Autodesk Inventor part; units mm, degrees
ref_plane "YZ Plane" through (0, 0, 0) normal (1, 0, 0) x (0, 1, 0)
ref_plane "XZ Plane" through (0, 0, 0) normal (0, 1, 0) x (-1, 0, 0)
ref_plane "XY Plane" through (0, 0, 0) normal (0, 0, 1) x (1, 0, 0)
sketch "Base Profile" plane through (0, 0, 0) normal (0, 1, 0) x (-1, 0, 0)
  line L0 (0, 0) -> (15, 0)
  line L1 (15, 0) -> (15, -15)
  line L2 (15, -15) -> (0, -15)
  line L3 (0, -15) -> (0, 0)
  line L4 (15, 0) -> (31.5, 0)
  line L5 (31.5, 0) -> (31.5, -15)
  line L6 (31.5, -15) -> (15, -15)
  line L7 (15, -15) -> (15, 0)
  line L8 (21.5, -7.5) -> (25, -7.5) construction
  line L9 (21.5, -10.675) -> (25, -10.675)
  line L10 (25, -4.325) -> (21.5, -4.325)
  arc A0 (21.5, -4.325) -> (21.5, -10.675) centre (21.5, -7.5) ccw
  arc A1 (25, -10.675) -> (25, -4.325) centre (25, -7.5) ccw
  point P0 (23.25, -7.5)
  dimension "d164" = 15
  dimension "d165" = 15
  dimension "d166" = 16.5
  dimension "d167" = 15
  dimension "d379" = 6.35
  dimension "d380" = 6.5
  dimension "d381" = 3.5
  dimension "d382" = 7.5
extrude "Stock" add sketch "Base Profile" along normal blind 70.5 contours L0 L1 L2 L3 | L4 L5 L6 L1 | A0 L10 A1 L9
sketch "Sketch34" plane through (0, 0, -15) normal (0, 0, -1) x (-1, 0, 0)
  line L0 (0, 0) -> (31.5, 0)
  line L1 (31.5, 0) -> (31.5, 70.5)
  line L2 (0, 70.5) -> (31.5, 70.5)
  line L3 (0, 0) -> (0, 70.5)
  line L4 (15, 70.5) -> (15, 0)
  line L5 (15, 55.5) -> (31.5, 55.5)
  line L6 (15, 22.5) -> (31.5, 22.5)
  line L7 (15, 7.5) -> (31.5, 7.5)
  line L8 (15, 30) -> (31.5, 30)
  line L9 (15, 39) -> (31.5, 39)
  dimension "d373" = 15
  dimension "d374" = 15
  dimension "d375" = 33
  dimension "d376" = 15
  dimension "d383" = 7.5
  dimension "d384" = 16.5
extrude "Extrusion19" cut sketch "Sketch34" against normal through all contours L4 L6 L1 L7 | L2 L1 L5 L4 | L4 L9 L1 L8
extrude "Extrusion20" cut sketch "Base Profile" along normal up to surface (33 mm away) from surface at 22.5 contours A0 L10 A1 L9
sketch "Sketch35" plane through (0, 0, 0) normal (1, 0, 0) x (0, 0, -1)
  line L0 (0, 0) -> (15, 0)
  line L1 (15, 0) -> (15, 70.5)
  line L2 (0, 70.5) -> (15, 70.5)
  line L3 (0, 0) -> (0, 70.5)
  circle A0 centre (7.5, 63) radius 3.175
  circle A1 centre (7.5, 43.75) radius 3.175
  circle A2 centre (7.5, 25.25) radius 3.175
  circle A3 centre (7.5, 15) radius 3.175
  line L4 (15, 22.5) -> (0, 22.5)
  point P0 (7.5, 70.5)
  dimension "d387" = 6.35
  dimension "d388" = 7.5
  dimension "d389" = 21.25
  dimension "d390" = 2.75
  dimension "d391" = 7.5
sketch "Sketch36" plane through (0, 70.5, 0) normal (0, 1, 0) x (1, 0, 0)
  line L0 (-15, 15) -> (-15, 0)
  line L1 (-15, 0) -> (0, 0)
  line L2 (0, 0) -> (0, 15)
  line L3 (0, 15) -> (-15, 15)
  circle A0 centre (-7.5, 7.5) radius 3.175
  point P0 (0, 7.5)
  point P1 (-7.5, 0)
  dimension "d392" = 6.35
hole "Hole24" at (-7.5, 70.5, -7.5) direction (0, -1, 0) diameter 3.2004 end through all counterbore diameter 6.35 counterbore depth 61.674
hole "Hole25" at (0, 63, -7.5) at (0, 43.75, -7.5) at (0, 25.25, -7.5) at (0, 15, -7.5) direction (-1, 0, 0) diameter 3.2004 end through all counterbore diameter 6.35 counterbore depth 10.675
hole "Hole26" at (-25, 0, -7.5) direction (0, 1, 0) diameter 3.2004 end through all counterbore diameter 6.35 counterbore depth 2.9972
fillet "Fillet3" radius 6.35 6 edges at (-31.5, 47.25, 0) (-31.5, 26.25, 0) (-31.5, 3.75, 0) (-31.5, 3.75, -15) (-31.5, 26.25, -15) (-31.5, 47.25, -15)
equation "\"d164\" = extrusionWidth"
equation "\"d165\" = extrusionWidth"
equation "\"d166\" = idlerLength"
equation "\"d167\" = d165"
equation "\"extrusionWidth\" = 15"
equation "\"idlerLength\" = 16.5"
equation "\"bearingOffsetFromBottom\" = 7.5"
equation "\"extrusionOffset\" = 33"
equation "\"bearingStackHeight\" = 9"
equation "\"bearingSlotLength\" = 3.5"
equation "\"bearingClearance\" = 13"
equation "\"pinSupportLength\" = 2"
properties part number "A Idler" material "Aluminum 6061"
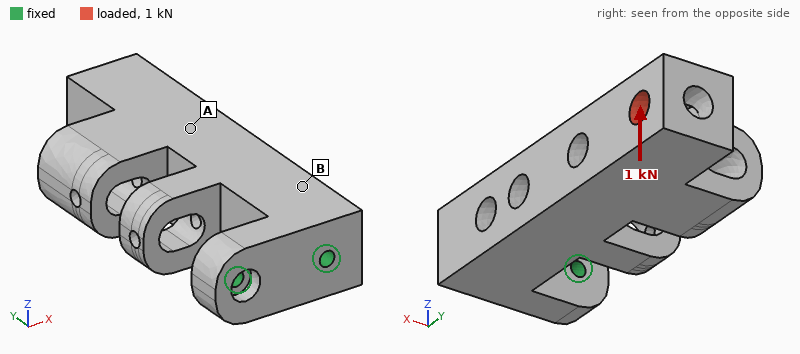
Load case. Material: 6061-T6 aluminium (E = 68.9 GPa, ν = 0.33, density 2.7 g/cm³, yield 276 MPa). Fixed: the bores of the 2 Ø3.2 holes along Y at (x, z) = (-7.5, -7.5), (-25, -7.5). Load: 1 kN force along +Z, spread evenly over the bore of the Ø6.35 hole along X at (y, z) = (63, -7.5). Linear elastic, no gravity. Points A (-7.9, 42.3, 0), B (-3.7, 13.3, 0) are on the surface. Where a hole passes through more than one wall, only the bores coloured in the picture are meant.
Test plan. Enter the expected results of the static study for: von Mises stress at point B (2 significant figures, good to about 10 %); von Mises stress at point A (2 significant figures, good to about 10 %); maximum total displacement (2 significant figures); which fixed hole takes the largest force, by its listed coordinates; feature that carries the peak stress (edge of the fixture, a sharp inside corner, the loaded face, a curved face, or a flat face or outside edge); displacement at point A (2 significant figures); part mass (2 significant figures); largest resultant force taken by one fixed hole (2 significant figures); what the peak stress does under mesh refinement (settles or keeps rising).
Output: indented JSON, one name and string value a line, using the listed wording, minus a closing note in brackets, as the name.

{
  "von Mises stress at point B": "96 MPa",
  "von Mises stress at point A": "45 MPa",
  "maximum total displacement": "0.52 mm",
  "which fixed hole takes the largest force, by its listed coordinates": "(-7.5, -7.5)",
  "feature that carries the peak stress": "edge of the fixture",
  "displacement at point A": "0.25 mm",
  "part mass": "51 g",
  "largest resultant force taken by one fixed hole": "1.2 kN",
  "what the peak stress does under mesh refinement": "keeps rising"
}
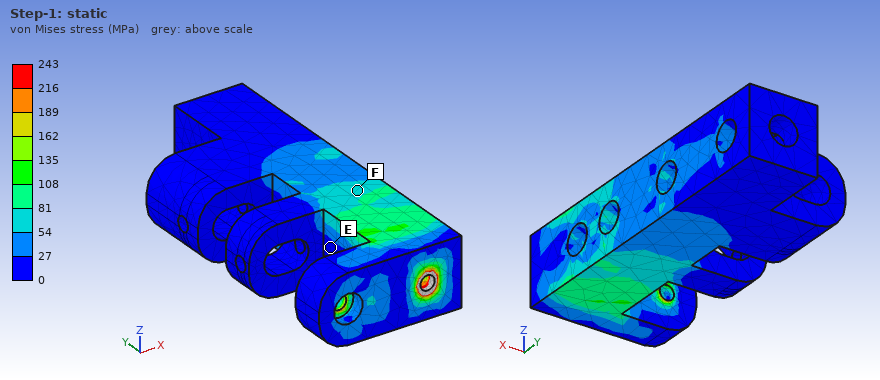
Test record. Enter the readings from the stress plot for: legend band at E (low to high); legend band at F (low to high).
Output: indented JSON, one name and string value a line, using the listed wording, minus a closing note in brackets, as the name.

{
  "legend band at E": "0 to 27 MPa",
  "legend band at F": "54 to 81 MPa"
}
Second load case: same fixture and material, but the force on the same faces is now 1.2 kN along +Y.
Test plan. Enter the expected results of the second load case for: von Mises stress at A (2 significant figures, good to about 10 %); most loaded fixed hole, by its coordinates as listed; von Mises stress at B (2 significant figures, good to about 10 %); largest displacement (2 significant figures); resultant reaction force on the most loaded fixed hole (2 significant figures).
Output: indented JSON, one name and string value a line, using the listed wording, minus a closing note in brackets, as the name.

{
  "von Mises stress at A": "5.7 MPa",
  "most loaded fixed hole, by its coordinates as listed": "(-7.5, -7.5)",
  "von Mises stress at B": "12 MPa",
  "largest displacement": "73 µm",
  "resultant reaction force on the most loaded fixed hole": "1.3 kN"
}
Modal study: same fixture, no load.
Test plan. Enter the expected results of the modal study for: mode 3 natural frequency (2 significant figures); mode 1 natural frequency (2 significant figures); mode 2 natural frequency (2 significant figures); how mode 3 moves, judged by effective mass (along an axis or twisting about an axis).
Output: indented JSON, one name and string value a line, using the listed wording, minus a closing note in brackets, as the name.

{
  "mode 3 natural frequency": "5500 Hz",
  "mode 1 natural frequency": "1900 Hz",
  "mode 2 natural frequency": "1900 Hz",
  "how mode 3 moves, judged by effective mass": "twisting about Y"
}
